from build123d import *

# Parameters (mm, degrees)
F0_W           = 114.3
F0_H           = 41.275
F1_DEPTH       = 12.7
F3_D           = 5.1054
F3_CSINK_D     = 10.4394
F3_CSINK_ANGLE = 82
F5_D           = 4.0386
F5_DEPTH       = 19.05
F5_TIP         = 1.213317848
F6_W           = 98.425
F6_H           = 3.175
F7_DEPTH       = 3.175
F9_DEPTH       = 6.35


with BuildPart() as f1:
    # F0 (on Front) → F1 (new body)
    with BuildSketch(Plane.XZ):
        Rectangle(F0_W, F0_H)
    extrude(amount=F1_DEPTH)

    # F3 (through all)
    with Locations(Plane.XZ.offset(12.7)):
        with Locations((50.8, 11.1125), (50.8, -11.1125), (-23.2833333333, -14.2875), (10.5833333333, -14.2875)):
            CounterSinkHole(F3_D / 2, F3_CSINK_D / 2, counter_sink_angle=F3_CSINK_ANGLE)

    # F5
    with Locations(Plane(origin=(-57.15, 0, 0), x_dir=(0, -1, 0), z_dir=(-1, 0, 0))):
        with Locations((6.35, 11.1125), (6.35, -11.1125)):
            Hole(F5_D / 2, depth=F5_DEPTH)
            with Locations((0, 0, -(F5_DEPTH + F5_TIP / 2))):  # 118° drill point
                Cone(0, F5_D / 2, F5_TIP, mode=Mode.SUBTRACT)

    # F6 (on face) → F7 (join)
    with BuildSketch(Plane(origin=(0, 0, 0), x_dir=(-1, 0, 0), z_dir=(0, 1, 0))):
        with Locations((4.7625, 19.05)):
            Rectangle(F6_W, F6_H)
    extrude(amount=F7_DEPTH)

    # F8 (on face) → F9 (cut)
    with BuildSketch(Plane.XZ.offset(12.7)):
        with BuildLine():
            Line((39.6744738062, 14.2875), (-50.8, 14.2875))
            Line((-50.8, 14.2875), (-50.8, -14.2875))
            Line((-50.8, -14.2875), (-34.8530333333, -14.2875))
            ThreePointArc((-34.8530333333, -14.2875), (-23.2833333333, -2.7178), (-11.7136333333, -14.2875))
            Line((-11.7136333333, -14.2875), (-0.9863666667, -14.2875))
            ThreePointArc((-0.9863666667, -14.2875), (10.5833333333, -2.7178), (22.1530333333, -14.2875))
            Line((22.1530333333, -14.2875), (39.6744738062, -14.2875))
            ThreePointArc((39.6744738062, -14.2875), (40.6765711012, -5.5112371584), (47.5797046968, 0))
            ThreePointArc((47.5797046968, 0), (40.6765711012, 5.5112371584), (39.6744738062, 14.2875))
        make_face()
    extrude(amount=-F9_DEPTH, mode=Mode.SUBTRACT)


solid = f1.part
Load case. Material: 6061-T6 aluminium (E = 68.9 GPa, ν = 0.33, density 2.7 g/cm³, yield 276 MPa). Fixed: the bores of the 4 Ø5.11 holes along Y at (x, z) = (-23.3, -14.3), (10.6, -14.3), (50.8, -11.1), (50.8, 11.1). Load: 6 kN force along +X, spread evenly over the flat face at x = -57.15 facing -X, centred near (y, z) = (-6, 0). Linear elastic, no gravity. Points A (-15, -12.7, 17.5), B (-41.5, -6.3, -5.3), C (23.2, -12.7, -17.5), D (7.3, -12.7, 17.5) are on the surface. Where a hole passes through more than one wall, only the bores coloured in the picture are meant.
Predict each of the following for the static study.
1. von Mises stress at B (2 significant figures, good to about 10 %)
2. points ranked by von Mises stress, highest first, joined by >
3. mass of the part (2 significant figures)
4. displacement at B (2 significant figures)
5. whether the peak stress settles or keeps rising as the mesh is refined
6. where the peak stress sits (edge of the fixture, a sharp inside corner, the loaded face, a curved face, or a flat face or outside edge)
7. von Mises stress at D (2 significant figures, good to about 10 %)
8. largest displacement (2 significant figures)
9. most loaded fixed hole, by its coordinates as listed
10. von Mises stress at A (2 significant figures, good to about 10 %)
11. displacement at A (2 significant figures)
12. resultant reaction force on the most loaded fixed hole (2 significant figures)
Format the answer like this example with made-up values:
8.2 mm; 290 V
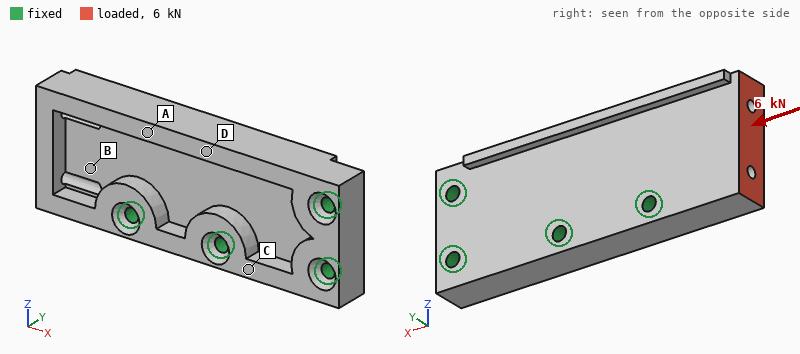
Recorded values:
38 MPa; B > A > D > C; 120 g; 17 µm; keeps rising; edge of the fixture; 17 MPa; 62 µm; (-23.3, -14.3); 27 MPa; 14 µm; 3.6 kN
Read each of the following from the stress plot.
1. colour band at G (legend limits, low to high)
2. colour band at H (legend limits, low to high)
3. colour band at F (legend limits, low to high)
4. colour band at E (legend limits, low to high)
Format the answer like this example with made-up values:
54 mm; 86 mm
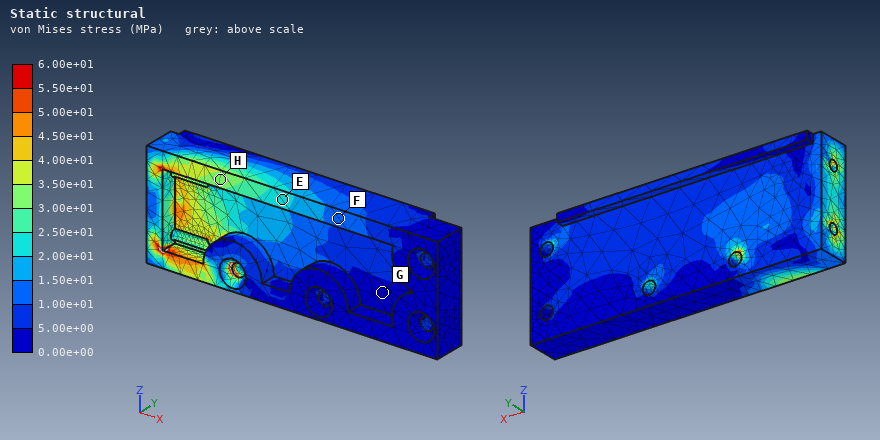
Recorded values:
0.00e+00 to 5.00e+00 MPa; 3.00e+01 to 3.50e+01 MPa; 1.00e+01 to 1.50e+01 MPa; 2.00e+01 to 2.50e+01 MPa
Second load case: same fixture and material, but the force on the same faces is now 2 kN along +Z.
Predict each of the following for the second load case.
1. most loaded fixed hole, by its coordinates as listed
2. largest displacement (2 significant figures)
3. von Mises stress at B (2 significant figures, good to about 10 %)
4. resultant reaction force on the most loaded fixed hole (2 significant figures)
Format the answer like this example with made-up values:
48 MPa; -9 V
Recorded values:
(-23.3, -14.3); 56 µm; 29 MPa; 3.2 kN
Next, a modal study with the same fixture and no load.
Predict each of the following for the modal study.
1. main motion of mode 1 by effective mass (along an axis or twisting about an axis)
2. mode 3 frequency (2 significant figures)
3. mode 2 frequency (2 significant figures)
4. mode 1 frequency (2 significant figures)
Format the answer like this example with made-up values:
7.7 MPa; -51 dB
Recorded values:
along Y; 8800 Hz; 6400 Hz; 3400 Hz
